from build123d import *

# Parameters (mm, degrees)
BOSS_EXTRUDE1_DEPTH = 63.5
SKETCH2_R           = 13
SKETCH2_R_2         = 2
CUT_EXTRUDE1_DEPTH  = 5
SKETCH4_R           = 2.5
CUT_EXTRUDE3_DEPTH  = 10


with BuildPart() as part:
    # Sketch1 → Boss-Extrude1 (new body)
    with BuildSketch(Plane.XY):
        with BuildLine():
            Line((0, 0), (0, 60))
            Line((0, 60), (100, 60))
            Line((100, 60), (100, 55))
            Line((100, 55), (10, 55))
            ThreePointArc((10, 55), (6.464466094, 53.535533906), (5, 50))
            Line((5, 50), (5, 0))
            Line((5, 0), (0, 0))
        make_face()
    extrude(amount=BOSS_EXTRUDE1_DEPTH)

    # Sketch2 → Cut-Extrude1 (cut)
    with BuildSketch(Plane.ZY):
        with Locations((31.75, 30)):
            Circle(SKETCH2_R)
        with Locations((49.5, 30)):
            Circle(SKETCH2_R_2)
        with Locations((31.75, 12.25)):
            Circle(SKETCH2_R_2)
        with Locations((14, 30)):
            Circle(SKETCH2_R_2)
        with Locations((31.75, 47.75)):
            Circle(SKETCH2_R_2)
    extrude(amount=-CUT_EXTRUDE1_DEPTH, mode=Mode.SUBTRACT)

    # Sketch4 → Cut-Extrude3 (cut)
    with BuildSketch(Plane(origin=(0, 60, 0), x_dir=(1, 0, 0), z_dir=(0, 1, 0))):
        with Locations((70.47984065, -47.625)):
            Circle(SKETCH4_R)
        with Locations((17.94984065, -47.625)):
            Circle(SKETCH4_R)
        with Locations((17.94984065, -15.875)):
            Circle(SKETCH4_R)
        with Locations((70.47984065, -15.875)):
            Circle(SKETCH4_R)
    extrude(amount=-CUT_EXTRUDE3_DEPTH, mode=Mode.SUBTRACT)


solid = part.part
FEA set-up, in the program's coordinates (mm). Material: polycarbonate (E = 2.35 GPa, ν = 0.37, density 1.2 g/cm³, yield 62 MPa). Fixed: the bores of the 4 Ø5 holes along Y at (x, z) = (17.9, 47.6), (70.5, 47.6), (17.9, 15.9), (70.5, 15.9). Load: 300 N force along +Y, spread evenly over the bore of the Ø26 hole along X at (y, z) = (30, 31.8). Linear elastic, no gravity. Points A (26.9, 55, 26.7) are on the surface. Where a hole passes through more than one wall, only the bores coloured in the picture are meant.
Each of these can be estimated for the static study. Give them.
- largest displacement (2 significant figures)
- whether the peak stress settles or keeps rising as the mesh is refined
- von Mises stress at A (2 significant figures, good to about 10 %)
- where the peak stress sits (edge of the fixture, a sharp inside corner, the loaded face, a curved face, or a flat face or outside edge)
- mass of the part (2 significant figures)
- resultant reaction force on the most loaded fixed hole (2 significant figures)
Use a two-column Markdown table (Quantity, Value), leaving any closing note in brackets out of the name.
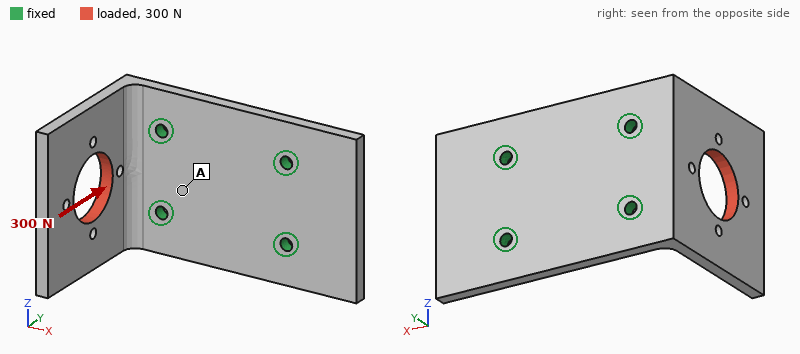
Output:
| Quantity | Value |
|---|---|
| largest displacement | 1.4 mm |
| whether the peak stress settles or keeps rising as the mesh is refined | keeps rising |
| von Mises stress at A | 2.1 MPa |
| where the peak stress sits | edge of the fixture |
| mass of the part | 56 g |
| resultant reaction force on the most loaded fixed hole | 160 N |
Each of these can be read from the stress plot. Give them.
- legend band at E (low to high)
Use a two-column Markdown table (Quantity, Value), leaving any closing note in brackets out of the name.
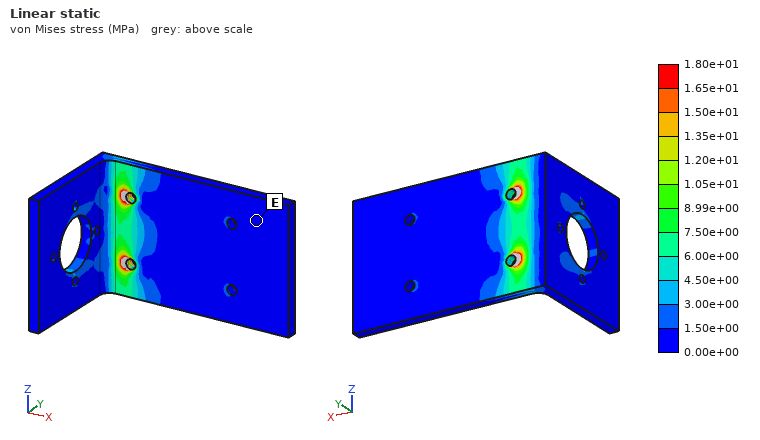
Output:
| Quantity | Value |
|---|---|
| legend band at E | 0.00e+00 to 1.50e+00 MPa |
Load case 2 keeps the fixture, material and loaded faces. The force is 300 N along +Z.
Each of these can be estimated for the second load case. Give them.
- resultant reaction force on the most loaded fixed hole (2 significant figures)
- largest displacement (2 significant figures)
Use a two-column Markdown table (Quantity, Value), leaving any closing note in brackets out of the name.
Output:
| Quantity | Value |
|---|---|
| resultant reaction force on the most loaded fixed hole | 290 N |
| largest displacement | 1.0 mm |
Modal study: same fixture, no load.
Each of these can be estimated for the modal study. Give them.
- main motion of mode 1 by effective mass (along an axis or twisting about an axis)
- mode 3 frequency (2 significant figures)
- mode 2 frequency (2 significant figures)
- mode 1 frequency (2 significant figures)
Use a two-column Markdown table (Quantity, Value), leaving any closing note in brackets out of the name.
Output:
| Quantity | Value |
|---|---|
| main motion of mode 1 by effective mass | along X |
| mode 3 frequency | 850 Hz |
| mode 2 frequency | 570 Hz |
| mode 1 frequency | 260 Hz |
